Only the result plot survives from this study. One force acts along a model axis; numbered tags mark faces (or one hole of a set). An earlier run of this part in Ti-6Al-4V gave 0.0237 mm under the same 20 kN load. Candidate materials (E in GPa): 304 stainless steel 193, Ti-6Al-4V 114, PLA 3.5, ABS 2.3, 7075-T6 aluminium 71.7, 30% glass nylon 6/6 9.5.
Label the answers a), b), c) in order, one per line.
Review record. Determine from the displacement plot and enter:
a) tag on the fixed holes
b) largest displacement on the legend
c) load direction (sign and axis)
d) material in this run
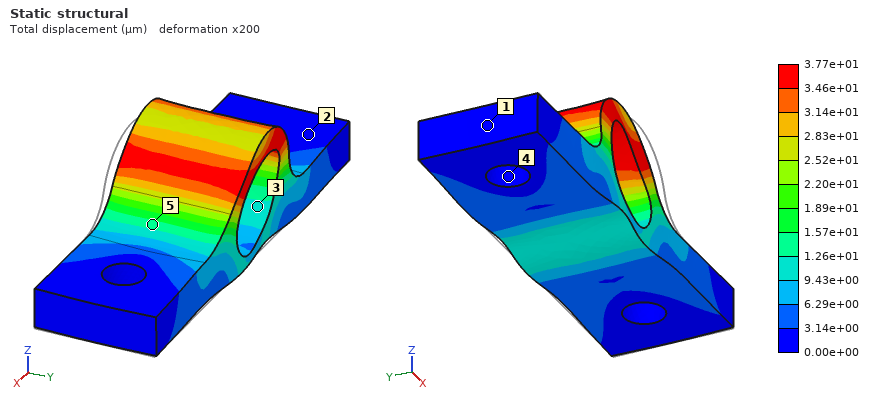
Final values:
a) 4
b) 3.77e+01 µm
c) -X
d) 7075-T6 aluminium
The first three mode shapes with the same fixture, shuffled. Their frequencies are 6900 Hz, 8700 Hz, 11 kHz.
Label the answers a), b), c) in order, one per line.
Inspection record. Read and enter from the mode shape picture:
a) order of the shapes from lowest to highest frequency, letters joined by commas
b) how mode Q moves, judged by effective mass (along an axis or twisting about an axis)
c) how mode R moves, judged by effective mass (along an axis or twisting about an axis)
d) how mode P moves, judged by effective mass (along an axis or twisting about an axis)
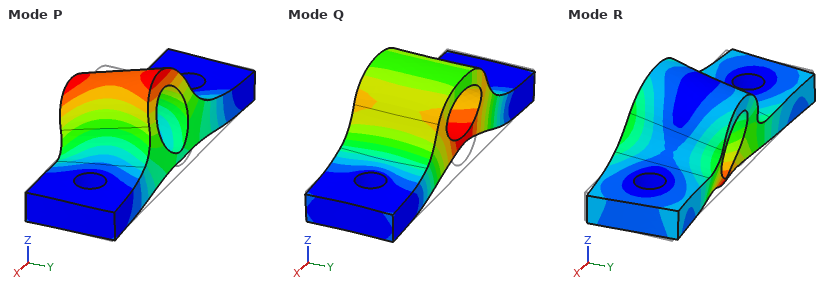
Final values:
a) P, Q, R
b) along Z
c) along Y
d) along Y
